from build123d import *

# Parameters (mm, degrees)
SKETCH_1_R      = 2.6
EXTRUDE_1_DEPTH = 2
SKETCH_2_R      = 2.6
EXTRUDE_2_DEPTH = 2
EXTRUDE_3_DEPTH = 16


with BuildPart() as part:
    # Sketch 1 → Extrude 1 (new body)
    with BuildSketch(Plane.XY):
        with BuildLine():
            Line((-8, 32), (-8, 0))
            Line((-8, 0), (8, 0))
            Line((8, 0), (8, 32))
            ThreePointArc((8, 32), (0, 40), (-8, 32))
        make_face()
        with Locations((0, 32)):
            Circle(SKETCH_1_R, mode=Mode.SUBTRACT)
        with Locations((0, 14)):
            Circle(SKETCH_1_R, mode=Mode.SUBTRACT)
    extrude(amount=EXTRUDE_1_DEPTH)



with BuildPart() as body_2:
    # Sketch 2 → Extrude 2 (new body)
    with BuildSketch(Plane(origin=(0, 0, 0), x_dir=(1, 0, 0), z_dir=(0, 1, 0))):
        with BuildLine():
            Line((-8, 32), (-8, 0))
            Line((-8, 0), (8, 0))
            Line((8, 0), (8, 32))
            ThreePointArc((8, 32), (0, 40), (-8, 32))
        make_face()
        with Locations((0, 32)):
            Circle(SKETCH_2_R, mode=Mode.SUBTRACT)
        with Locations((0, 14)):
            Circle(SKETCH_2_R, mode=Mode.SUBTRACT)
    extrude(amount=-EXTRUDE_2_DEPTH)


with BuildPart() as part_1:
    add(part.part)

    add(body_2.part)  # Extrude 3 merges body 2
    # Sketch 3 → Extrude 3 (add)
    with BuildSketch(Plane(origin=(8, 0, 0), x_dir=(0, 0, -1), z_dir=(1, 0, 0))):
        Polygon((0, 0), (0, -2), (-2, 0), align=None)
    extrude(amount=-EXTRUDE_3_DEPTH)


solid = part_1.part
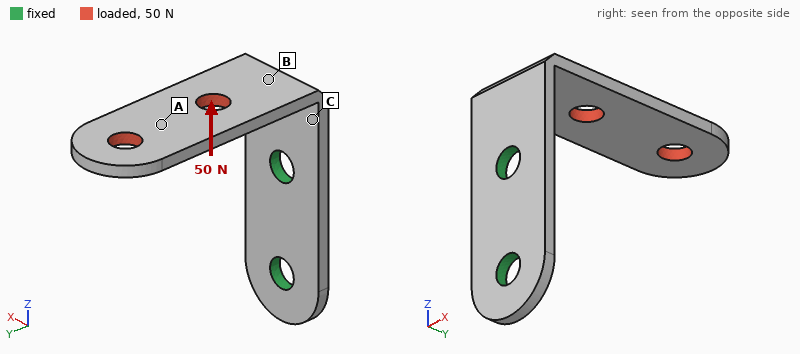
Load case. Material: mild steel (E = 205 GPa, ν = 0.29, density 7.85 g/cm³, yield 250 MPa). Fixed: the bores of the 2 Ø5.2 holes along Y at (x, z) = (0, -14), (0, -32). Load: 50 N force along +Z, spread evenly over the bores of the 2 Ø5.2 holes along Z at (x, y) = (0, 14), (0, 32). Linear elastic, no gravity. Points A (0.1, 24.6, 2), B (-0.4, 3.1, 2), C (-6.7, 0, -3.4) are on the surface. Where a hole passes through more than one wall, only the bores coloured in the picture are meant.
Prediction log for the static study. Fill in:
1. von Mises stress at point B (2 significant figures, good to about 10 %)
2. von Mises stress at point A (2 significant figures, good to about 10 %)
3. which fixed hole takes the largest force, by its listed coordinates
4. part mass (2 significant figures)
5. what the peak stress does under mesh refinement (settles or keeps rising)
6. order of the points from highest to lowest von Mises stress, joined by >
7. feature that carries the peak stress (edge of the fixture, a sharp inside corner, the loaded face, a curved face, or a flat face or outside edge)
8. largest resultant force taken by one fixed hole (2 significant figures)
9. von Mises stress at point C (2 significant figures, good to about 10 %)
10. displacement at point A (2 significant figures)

85 MPa
20 MPa
(0, -14)
18 g
keeps rising
C > B > A
edge of the fixture
46 N
110 MPa
0.32 mm
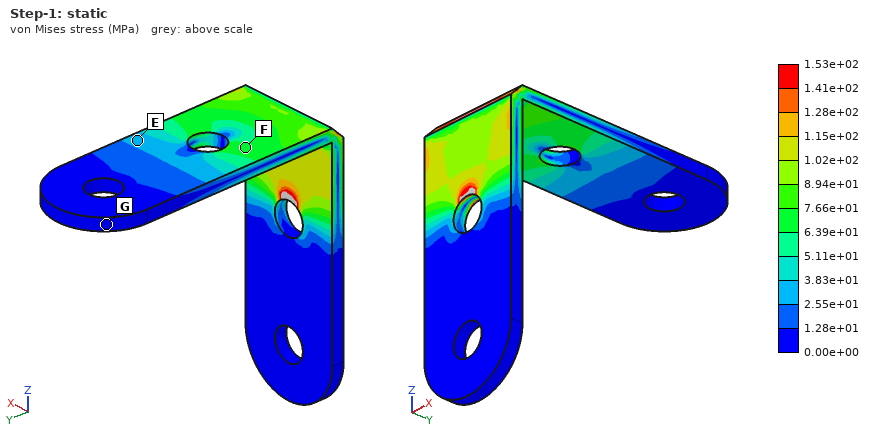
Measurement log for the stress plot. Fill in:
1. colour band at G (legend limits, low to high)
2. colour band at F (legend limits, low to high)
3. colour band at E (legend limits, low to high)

0.00e+00 to 1.28e+01 MPa
6.39e+01 to 7.66e+01 MPa
2.55e+01 to 3.83e+01 MPa
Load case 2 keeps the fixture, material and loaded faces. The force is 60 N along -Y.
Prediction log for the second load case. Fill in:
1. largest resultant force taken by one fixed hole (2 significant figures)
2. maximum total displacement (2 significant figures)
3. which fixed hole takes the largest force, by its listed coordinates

62 N
0.10 mm
(0, -14)
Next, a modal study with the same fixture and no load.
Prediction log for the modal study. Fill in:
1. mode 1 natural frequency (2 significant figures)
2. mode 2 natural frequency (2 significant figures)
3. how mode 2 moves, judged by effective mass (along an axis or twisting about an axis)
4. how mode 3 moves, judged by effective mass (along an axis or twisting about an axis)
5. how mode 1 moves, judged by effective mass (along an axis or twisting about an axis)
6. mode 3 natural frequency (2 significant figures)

700 Hz
1200 Hz
along X
along Y
along Z
3200 Hz
